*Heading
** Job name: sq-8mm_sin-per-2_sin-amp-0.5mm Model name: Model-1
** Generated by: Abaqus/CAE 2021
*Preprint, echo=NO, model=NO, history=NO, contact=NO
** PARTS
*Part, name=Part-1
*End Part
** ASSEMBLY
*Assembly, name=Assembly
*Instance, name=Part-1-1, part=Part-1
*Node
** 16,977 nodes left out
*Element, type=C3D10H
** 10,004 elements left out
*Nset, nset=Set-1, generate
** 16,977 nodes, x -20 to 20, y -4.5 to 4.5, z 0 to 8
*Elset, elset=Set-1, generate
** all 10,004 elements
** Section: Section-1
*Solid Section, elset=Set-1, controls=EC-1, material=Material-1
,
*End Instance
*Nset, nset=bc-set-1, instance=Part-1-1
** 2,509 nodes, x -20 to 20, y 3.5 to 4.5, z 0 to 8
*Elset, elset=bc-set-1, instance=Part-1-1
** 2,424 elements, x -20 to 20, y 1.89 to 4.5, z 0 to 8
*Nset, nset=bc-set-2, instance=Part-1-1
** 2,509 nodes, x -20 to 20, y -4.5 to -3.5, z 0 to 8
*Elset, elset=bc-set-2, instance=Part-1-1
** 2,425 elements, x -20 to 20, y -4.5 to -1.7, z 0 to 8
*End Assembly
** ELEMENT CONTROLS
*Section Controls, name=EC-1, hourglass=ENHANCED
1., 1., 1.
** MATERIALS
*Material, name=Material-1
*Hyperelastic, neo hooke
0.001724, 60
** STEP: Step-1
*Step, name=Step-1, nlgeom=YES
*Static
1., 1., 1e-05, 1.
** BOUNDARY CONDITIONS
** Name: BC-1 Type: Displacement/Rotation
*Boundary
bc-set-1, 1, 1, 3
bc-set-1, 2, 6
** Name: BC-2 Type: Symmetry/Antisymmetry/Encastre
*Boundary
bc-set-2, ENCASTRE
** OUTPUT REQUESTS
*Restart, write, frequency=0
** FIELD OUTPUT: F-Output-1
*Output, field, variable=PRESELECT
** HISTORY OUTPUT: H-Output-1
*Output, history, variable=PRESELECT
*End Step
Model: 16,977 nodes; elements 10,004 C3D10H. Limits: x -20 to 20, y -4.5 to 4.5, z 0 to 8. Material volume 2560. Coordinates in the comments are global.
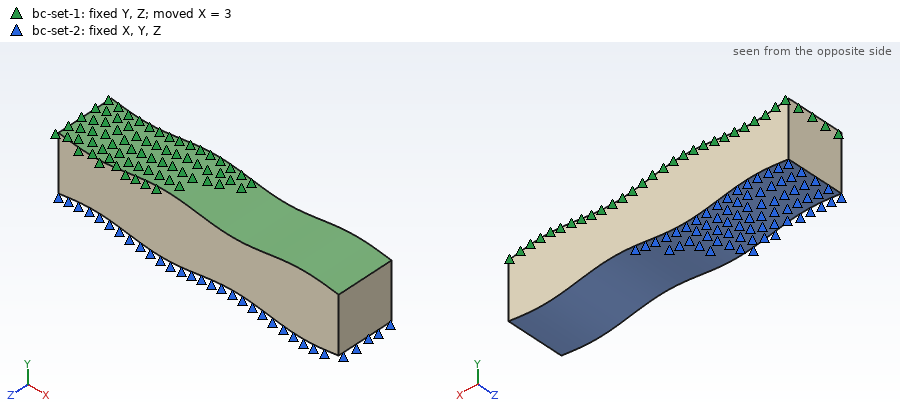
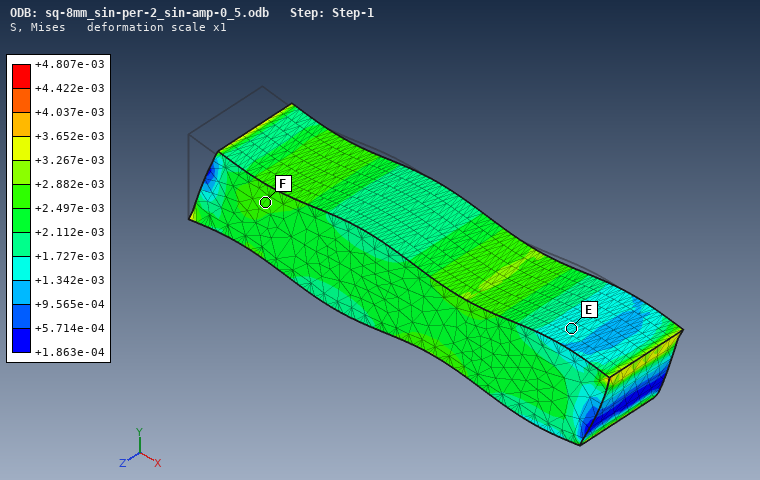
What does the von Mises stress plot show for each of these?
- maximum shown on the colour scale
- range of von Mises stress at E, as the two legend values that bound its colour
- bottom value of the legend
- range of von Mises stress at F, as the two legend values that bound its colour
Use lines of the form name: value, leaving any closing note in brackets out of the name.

maximum shown on the colour scale: +4.807e-03
range of von Mises stress at E, as the two legend values that bound its colour: +1.342e-03 to +1.727e-03
bottom value of the legend: +1.863e-04
range of von Mises stress at F, as the two legend values that bound its colour: +2.497e-03 to +2.882e-03
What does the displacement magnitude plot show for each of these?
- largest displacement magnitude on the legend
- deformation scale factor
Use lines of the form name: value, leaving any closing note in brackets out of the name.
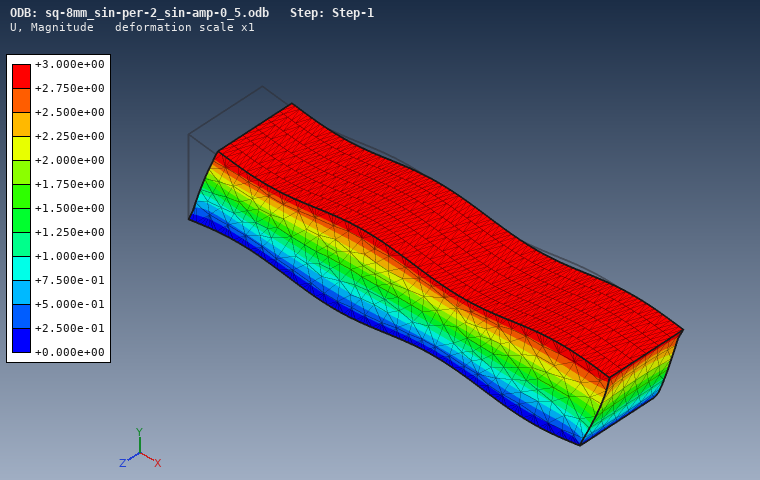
largest displacement magnitude on the legend: +3.000e+00
deformation scale factor: 1
